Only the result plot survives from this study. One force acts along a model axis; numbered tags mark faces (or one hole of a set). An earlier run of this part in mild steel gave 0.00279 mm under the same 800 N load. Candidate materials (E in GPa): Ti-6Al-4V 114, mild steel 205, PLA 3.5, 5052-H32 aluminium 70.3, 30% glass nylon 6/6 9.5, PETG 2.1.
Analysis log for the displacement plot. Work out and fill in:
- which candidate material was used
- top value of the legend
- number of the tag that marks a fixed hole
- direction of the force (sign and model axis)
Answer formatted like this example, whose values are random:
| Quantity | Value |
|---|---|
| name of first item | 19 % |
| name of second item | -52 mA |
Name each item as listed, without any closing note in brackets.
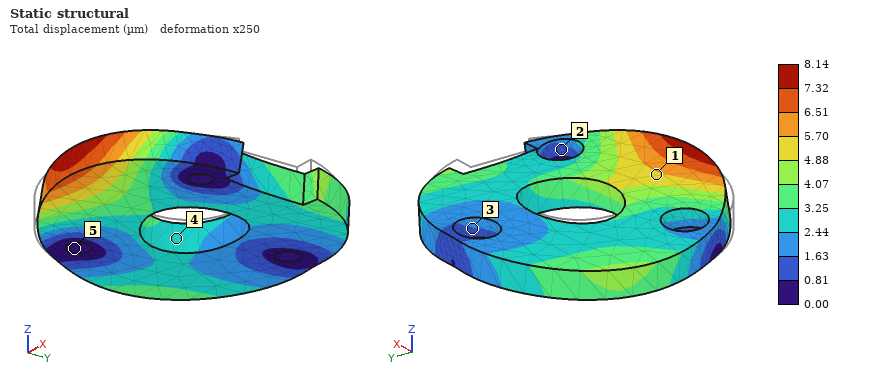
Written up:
| Quantity | Value |
|---|---|
| which candidate material was used | 5052-H32 aluminium |
| top value of the legend | 8.14 µm |
| number of the tag that marks a fixed hole | 5 |
| direction of the force | +Y |
